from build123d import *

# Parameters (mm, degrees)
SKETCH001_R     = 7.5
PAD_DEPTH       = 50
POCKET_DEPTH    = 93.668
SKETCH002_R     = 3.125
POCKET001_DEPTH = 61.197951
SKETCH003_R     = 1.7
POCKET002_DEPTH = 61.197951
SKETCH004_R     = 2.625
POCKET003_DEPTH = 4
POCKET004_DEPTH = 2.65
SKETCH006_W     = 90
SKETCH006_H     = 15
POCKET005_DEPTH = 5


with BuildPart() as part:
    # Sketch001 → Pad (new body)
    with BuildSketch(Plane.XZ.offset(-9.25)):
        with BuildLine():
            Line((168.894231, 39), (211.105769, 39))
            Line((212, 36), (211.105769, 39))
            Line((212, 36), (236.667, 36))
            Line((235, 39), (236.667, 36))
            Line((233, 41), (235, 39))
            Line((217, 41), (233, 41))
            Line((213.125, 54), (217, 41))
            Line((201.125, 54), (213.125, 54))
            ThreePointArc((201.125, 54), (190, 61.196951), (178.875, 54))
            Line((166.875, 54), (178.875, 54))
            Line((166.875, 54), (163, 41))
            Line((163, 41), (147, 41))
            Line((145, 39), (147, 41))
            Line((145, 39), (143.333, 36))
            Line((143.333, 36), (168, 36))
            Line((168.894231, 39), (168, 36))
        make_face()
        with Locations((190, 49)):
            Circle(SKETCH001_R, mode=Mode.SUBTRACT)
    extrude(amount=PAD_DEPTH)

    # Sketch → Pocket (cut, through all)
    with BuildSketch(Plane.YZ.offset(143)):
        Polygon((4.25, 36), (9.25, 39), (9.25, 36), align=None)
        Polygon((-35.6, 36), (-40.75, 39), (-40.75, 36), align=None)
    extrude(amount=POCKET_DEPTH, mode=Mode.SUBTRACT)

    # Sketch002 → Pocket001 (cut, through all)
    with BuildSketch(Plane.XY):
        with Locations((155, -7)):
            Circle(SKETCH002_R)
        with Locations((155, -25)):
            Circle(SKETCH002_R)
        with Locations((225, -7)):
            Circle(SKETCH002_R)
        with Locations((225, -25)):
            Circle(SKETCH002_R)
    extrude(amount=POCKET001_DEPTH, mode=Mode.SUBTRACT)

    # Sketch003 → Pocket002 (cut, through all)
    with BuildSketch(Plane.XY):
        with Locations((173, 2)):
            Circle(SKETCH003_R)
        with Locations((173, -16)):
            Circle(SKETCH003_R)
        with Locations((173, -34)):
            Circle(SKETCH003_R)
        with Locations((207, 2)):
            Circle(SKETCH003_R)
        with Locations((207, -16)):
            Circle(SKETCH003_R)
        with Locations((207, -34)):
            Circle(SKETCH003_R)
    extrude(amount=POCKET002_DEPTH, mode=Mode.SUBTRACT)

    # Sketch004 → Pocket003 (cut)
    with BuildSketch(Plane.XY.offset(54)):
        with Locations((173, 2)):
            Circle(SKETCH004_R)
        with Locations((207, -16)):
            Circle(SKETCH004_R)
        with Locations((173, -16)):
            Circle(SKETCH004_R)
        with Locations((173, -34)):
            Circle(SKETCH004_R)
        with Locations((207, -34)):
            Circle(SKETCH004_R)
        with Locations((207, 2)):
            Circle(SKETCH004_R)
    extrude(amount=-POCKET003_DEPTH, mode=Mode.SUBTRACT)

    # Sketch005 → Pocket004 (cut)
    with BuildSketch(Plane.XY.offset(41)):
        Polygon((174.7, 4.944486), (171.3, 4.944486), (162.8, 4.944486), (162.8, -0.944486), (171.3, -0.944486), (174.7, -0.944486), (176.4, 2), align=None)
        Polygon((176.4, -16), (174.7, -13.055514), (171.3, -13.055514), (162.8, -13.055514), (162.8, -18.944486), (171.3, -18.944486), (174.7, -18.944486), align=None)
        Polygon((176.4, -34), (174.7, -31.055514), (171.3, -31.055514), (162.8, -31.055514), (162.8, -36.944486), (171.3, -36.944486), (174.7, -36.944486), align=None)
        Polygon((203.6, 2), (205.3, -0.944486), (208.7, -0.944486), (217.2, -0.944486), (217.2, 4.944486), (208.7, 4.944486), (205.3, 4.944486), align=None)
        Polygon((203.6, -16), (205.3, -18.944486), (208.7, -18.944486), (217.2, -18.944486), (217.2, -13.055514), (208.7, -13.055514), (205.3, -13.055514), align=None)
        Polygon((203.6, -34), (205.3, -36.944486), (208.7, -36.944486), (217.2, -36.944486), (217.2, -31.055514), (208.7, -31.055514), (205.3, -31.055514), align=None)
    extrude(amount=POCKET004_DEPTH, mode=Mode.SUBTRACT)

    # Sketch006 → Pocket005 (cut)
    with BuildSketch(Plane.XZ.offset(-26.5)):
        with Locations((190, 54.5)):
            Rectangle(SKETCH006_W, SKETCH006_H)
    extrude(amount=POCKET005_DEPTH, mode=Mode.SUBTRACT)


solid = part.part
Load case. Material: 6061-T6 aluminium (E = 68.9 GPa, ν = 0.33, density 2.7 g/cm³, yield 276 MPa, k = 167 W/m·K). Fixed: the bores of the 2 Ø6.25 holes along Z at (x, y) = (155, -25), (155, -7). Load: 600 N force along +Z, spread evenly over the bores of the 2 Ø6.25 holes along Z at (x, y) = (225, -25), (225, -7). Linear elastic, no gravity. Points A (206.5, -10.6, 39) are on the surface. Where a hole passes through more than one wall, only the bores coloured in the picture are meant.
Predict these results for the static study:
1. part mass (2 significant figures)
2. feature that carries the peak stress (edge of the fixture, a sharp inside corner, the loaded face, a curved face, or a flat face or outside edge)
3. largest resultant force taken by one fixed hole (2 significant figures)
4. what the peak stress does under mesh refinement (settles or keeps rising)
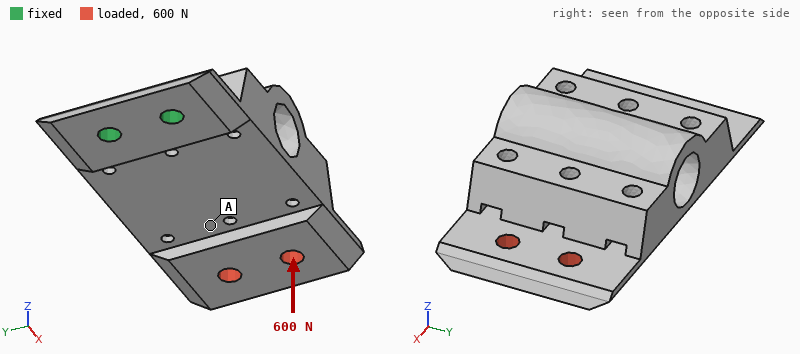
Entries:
110 g
edge of the fixture
310 N
keeps rising
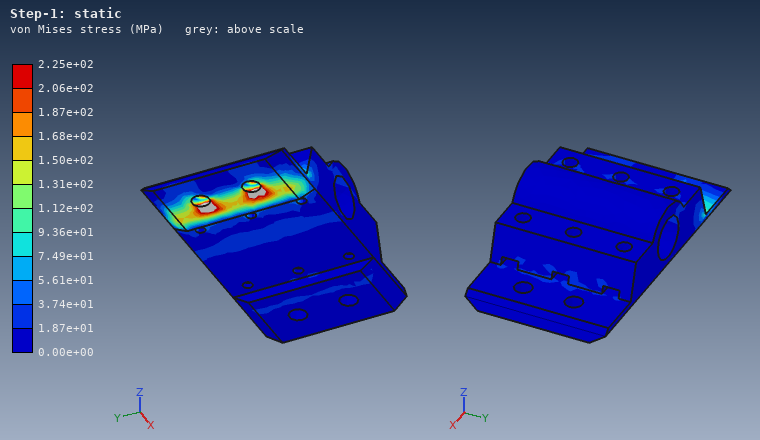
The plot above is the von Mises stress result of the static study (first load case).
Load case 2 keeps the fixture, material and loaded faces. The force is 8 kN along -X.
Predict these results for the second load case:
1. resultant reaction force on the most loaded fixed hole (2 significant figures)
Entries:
4.0 kN
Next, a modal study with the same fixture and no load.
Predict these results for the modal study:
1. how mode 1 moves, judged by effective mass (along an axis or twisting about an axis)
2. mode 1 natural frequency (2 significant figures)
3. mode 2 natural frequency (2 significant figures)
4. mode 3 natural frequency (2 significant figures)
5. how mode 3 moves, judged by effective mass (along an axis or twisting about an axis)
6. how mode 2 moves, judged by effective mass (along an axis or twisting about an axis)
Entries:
along Z
680 Hz
2800 Hz
3600 Hz
along Y
along Y
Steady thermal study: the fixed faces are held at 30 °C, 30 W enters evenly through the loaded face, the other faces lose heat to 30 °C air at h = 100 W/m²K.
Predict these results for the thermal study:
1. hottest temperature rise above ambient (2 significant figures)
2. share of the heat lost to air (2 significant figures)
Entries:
28 K
57 %
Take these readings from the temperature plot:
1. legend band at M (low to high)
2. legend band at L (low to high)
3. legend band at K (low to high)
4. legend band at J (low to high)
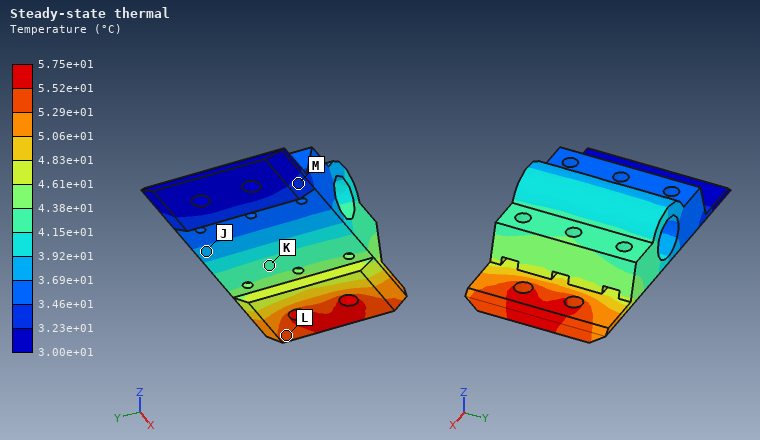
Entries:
3.23e+01 to 3.46e+01 °C
5.29e+01 to 5.52e+01 °C
4.15e+01 to 4.38e+01 °C
3.69e+01 to 3.92e+01 °C
